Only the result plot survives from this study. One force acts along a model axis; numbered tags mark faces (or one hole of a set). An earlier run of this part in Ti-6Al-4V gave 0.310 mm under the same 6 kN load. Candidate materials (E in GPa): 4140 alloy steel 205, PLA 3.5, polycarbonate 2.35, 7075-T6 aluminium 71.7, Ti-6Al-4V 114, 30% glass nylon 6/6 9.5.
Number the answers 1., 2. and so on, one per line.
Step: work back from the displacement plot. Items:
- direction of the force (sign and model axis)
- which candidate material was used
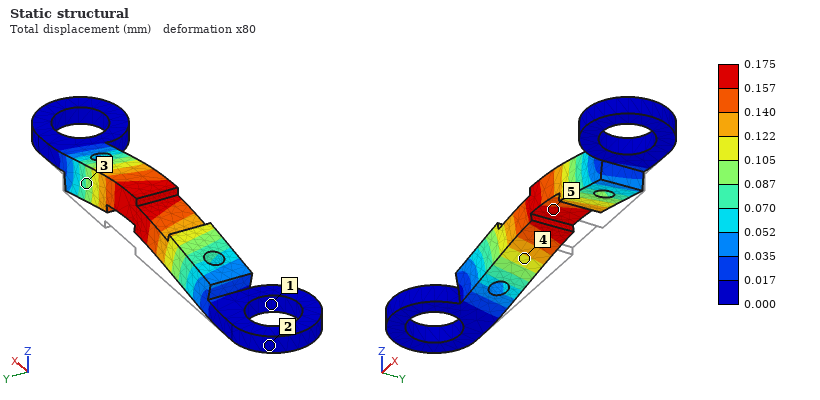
1. +Z
2. 4140 alloy steel
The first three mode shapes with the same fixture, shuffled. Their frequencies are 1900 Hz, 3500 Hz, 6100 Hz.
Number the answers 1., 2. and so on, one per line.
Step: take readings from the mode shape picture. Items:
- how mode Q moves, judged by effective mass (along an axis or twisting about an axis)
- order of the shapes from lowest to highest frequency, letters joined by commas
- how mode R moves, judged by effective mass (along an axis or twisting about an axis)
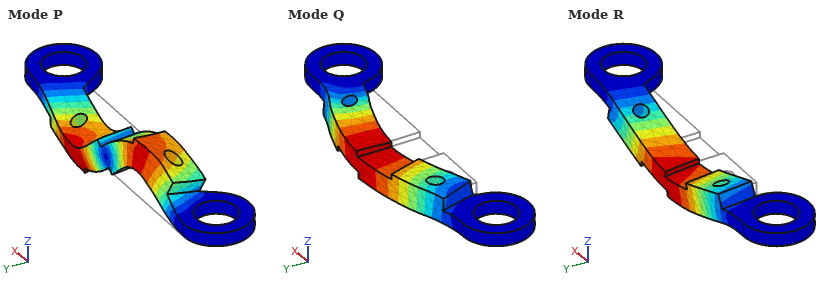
1. along Y
2. R, Q, P
3. along Z
